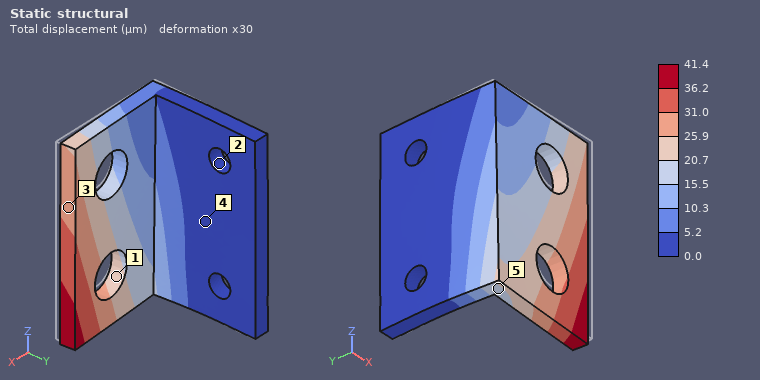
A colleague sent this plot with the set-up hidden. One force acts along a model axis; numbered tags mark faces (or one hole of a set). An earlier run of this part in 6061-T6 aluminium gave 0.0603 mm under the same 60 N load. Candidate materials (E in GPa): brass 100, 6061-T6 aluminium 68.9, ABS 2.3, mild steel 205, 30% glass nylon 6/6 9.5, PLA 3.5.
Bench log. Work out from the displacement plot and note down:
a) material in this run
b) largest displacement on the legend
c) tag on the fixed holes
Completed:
brass
41.4 µm
2
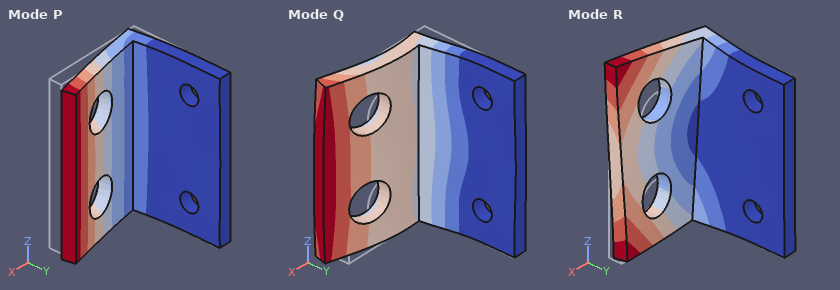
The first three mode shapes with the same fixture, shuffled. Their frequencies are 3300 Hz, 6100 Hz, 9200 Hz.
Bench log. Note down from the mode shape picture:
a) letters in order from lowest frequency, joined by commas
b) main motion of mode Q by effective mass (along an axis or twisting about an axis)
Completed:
P, R, Q
along X
